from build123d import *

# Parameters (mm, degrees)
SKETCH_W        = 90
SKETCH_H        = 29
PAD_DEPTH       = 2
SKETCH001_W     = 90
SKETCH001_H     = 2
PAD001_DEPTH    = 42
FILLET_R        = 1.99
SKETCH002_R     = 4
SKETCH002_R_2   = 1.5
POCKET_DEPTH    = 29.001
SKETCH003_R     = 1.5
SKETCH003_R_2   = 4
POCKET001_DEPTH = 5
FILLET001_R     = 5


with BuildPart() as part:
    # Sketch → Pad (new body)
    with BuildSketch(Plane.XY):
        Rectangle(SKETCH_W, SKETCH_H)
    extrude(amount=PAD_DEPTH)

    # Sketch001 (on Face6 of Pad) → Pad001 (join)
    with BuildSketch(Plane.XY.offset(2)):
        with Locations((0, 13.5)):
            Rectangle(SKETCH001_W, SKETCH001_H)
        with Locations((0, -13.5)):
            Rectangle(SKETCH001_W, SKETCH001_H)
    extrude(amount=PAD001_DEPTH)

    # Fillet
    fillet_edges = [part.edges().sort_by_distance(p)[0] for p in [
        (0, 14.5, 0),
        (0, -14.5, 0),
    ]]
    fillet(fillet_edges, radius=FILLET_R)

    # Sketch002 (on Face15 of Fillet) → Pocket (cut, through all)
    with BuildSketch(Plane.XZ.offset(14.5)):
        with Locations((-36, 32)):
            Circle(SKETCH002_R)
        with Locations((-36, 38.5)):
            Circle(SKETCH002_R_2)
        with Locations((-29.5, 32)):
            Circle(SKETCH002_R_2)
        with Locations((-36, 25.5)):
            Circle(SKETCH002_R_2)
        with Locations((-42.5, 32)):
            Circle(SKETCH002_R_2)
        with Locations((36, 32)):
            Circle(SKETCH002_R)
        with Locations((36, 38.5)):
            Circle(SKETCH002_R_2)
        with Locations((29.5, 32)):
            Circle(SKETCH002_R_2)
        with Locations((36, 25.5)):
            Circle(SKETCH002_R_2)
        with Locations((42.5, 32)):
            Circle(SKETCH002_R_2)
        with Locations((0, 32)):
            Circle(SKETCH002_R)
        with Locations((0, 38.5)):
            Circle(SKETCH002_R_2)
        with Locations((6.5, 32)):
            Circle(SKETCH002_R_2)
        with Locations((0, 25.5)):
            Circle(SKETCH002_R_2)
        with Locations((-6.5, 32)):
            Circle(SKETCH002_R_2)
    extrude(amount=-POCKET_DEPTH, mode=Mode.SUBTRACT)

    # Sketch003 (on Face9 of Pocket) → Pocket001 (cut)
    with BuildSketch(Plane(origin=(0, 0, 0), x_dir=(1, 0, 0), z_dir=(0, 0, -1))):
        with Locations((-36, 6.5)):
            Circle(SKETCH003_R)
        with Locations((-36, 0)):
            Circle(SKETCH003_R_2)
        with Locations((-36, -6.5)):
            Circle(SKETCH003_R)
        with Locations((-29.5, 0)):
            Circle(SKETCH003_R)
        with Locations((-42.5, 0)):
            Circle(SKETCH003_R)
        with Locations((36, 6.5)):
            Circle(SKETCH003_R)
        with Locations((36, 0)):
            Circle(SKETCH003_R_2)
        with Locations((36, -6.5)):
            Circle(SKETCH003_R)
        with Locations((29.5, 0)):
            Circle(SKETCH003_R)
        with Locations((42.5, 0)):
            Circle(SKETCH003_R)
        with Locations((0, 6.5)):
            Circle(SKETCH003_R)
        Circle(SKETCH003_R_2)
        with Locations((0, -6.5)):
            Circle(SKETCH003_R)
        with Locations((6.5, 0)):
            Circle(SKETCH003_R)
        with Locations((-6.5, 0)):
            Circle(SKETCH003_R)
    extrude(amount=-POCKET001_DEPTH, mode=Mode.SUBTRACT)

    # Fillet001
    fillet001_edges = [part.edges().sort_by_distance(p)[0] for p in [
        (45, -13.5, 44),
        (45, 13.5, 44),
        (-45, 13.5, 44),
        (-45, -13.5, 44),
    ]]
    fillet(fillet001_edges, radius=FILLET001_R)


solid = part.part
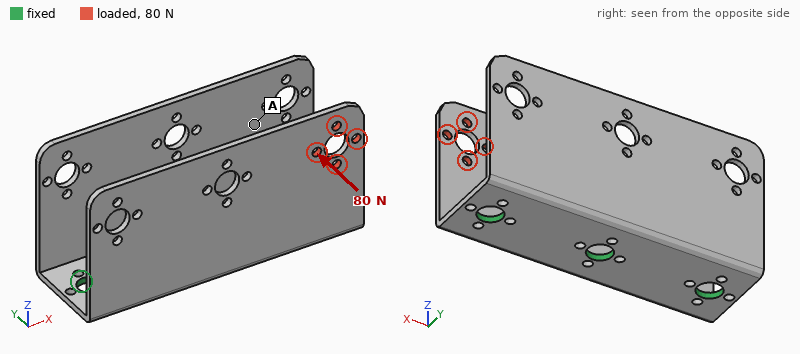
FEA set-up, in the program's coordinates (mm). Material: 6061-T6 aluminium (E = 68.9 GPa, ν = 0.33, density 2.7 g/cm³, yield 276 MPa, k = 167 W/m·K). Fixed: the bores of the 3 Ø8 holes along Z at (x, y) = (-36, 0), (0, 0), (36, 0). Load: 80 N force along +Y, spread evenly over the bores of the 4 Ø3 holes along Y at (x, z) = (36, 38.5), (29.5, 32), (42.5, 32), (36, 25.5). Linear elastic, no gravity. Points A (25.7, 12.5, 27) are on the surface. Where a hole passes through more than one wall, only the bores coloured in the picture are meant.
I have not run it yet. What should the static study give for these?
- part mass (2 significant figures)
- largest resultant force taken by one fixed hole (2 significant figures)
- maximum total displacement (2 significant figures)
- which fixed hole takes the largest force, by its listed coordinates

51 g
70 N
1.0 mm
(36, 0)
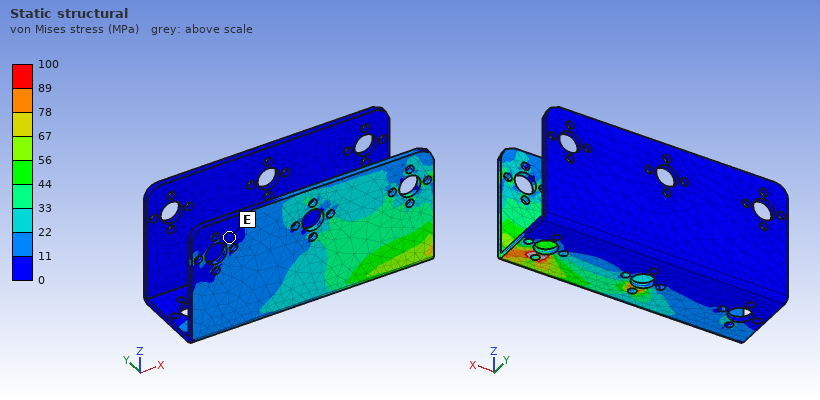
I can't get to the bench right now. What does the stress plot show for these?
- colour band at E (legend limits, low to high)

0 to 11 MPa
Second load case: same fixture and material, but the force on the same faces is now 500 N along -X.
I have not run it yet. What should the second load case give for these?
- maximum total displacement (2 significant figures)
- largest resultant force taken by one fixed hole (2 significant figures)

0.26 mm
270 N
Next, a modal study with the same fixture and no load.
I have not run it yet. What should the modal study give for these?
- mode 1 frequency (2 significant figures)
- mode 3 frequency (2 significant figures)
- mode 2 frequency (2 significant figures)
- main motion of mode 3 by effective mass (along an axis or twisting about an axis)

650 Hz
1100 Hz
660 Hz
twisting about Z
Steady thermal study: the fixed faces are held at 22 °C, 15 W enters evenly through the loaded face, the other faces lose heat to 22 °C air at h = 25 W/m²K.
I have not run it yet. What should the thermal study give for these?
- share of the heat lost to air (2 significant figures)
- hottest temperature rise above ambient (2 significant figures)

22 %
50 K
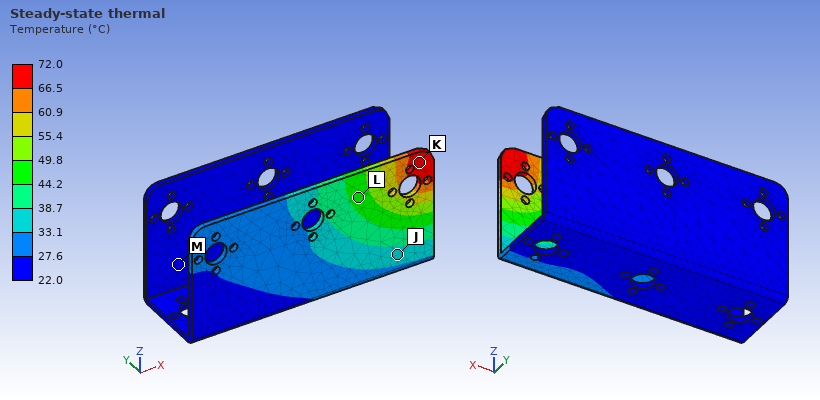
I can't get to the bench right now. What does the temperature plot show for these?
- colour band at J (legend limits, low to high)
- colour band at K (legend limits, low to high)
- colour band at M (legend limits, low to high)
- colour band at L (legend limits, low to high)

33.1 to 38.7 °C
66.5 to 72.0 °C
22.0 to 27.6 °C
44.2 to 49.8 °C
